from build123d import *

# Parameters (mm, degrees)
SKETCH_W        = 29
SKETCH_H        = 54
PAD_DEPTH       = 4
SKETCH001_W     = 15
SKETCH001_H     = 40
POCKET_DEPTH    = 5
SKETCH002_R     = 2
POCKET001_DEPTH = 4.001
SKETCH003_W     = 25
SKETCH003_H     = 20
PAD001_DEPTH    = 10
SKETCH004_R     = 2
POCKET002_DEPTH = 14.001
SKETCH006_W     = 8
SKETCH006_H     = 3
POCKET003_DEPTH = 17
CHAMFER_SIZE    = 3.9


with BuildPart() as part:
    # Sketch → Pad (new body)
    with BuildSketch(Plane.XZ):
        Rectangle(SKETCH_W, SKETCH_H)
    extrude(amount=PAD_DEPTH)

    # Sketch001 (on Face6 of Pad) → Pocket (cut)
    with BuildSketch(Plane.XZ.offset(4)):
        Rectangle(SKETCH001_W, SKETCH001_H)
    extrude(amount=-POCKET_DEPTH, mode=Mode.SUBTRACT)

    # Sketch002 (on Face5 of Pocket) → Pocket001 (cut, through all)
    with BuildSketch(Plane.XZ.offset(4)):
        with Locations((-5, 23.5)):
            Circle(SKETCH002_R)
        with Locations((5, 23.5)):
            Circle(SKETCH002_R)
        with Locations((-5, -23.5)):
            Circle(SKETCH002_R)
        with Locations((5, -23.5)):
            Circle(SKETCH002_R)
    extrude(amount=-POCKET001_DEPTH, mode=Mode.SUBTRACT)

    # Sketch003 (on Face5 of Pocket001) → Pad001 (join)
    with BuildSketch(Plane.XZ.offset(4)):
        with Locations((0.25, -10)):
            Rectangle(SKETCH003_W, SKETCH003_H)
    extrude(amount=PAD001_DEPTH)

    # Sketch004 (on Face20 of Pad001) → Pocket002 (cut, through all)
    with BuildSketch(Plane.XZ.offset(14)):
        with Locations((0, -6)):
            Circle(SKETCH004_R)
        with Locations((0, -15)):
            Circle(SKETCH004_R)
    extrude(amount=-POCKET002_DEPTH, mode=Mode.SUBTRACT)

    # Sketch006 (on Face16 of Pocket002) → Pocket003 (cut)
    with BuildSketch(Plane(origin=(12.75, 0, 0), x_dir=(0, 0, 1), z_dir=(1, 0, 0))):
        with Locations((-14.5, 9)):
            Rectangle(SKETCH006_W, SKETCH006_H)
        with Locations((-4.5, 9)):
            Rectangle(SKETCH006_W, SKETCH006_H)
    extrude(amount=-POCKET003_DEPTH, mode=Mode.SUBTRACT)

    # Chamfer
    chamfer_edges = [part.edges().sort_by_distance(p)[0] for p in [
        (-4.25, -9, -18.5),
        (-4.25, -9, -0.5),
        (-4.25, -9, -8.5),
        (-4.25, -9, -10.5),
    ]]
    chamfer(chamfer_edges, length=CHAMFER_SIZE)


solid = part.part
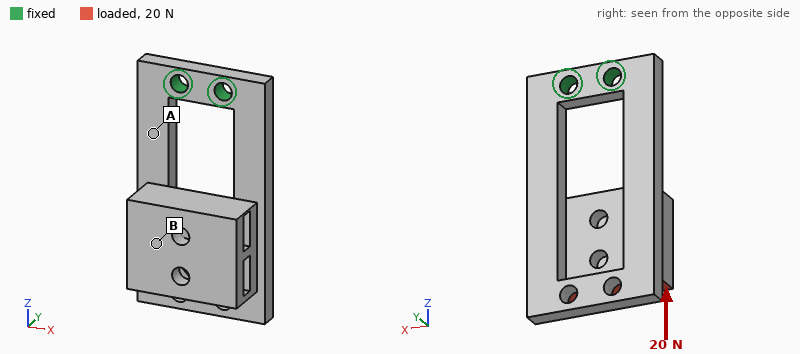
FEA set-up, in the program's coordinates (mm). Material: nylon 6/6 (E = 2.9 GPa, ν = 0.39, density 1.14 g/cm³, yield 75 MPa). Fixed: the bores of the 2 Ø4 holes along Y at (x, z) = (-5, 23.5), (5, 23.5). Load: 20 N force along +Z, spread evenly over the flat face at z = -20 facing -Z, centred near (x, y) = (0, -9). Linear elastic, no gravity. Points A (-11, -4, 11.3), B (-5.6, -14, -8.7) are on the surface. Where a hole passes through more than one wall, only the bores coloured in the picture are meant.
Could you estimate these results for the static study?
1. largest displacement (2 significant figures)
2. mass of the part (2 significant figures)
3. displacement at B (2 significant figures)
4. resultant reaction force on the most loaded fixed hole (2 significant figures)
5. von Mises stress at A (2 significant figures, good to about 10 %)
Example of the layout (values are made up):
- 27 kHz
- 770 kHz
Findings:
- 0.68 mm
- 8.8 g
- 0.41 mm
- 10 N
- 4.1 MPa
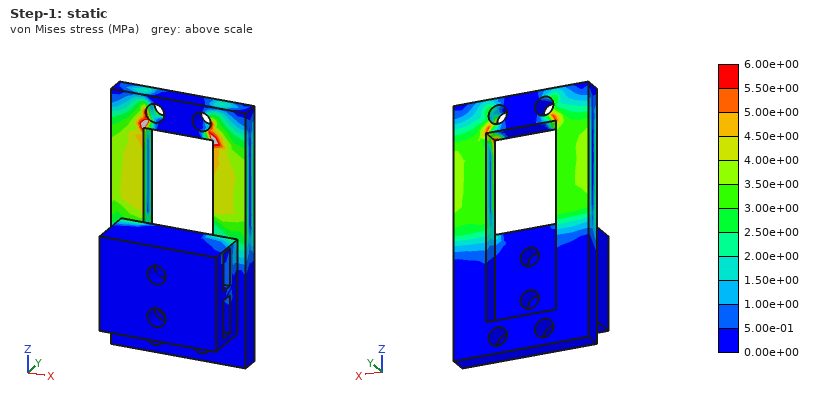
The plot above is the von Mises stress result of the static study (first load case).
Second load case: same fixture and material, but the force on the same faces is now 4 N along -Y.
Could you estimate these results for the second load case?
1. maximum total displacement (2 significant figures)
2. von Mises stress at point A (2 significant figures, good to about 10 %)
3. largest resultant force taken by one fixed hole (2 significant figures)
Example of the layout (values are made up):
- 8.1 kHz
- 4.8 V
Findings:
- 0.64 mm
- 3.3 MPa
- 2.1 N
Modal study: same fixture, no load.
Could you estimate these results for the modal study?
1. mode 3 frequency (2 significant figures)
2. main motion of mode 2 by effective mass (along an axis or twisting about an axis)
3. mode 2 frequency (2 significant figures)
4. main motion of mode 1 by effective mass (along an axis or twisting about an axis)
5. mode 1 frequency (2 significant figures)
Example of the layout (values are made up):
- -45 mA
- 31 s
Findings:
- 900 Hz
- along X
- 630 Hz
- along Y
- 210 Hz
